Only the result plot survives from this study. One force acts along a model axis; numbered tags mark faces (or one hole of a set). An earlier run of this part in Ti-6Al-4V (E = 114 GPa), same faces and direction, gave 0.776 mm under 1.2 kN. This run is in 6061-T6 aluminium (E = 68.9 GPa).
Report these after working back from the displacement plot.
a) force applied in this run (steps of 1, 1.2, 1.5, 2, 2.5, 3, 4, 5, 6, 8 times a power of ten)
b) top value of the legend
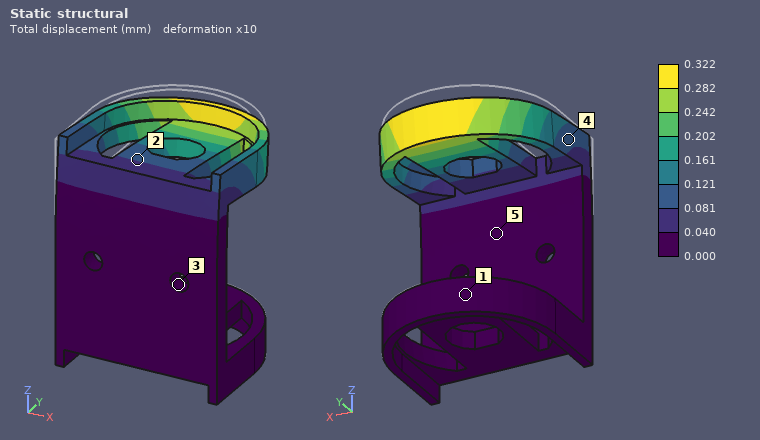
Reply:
300 N
0.322 mm
